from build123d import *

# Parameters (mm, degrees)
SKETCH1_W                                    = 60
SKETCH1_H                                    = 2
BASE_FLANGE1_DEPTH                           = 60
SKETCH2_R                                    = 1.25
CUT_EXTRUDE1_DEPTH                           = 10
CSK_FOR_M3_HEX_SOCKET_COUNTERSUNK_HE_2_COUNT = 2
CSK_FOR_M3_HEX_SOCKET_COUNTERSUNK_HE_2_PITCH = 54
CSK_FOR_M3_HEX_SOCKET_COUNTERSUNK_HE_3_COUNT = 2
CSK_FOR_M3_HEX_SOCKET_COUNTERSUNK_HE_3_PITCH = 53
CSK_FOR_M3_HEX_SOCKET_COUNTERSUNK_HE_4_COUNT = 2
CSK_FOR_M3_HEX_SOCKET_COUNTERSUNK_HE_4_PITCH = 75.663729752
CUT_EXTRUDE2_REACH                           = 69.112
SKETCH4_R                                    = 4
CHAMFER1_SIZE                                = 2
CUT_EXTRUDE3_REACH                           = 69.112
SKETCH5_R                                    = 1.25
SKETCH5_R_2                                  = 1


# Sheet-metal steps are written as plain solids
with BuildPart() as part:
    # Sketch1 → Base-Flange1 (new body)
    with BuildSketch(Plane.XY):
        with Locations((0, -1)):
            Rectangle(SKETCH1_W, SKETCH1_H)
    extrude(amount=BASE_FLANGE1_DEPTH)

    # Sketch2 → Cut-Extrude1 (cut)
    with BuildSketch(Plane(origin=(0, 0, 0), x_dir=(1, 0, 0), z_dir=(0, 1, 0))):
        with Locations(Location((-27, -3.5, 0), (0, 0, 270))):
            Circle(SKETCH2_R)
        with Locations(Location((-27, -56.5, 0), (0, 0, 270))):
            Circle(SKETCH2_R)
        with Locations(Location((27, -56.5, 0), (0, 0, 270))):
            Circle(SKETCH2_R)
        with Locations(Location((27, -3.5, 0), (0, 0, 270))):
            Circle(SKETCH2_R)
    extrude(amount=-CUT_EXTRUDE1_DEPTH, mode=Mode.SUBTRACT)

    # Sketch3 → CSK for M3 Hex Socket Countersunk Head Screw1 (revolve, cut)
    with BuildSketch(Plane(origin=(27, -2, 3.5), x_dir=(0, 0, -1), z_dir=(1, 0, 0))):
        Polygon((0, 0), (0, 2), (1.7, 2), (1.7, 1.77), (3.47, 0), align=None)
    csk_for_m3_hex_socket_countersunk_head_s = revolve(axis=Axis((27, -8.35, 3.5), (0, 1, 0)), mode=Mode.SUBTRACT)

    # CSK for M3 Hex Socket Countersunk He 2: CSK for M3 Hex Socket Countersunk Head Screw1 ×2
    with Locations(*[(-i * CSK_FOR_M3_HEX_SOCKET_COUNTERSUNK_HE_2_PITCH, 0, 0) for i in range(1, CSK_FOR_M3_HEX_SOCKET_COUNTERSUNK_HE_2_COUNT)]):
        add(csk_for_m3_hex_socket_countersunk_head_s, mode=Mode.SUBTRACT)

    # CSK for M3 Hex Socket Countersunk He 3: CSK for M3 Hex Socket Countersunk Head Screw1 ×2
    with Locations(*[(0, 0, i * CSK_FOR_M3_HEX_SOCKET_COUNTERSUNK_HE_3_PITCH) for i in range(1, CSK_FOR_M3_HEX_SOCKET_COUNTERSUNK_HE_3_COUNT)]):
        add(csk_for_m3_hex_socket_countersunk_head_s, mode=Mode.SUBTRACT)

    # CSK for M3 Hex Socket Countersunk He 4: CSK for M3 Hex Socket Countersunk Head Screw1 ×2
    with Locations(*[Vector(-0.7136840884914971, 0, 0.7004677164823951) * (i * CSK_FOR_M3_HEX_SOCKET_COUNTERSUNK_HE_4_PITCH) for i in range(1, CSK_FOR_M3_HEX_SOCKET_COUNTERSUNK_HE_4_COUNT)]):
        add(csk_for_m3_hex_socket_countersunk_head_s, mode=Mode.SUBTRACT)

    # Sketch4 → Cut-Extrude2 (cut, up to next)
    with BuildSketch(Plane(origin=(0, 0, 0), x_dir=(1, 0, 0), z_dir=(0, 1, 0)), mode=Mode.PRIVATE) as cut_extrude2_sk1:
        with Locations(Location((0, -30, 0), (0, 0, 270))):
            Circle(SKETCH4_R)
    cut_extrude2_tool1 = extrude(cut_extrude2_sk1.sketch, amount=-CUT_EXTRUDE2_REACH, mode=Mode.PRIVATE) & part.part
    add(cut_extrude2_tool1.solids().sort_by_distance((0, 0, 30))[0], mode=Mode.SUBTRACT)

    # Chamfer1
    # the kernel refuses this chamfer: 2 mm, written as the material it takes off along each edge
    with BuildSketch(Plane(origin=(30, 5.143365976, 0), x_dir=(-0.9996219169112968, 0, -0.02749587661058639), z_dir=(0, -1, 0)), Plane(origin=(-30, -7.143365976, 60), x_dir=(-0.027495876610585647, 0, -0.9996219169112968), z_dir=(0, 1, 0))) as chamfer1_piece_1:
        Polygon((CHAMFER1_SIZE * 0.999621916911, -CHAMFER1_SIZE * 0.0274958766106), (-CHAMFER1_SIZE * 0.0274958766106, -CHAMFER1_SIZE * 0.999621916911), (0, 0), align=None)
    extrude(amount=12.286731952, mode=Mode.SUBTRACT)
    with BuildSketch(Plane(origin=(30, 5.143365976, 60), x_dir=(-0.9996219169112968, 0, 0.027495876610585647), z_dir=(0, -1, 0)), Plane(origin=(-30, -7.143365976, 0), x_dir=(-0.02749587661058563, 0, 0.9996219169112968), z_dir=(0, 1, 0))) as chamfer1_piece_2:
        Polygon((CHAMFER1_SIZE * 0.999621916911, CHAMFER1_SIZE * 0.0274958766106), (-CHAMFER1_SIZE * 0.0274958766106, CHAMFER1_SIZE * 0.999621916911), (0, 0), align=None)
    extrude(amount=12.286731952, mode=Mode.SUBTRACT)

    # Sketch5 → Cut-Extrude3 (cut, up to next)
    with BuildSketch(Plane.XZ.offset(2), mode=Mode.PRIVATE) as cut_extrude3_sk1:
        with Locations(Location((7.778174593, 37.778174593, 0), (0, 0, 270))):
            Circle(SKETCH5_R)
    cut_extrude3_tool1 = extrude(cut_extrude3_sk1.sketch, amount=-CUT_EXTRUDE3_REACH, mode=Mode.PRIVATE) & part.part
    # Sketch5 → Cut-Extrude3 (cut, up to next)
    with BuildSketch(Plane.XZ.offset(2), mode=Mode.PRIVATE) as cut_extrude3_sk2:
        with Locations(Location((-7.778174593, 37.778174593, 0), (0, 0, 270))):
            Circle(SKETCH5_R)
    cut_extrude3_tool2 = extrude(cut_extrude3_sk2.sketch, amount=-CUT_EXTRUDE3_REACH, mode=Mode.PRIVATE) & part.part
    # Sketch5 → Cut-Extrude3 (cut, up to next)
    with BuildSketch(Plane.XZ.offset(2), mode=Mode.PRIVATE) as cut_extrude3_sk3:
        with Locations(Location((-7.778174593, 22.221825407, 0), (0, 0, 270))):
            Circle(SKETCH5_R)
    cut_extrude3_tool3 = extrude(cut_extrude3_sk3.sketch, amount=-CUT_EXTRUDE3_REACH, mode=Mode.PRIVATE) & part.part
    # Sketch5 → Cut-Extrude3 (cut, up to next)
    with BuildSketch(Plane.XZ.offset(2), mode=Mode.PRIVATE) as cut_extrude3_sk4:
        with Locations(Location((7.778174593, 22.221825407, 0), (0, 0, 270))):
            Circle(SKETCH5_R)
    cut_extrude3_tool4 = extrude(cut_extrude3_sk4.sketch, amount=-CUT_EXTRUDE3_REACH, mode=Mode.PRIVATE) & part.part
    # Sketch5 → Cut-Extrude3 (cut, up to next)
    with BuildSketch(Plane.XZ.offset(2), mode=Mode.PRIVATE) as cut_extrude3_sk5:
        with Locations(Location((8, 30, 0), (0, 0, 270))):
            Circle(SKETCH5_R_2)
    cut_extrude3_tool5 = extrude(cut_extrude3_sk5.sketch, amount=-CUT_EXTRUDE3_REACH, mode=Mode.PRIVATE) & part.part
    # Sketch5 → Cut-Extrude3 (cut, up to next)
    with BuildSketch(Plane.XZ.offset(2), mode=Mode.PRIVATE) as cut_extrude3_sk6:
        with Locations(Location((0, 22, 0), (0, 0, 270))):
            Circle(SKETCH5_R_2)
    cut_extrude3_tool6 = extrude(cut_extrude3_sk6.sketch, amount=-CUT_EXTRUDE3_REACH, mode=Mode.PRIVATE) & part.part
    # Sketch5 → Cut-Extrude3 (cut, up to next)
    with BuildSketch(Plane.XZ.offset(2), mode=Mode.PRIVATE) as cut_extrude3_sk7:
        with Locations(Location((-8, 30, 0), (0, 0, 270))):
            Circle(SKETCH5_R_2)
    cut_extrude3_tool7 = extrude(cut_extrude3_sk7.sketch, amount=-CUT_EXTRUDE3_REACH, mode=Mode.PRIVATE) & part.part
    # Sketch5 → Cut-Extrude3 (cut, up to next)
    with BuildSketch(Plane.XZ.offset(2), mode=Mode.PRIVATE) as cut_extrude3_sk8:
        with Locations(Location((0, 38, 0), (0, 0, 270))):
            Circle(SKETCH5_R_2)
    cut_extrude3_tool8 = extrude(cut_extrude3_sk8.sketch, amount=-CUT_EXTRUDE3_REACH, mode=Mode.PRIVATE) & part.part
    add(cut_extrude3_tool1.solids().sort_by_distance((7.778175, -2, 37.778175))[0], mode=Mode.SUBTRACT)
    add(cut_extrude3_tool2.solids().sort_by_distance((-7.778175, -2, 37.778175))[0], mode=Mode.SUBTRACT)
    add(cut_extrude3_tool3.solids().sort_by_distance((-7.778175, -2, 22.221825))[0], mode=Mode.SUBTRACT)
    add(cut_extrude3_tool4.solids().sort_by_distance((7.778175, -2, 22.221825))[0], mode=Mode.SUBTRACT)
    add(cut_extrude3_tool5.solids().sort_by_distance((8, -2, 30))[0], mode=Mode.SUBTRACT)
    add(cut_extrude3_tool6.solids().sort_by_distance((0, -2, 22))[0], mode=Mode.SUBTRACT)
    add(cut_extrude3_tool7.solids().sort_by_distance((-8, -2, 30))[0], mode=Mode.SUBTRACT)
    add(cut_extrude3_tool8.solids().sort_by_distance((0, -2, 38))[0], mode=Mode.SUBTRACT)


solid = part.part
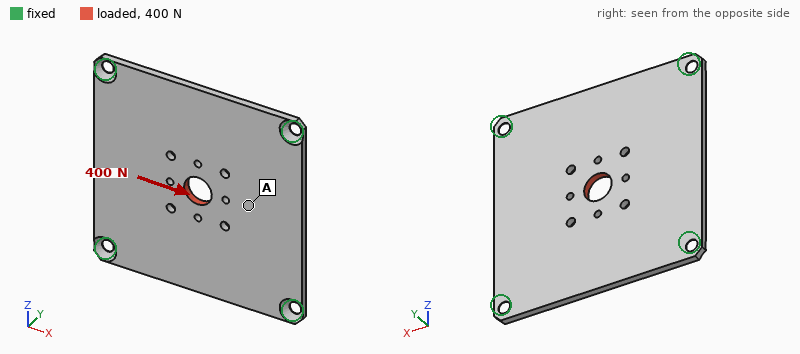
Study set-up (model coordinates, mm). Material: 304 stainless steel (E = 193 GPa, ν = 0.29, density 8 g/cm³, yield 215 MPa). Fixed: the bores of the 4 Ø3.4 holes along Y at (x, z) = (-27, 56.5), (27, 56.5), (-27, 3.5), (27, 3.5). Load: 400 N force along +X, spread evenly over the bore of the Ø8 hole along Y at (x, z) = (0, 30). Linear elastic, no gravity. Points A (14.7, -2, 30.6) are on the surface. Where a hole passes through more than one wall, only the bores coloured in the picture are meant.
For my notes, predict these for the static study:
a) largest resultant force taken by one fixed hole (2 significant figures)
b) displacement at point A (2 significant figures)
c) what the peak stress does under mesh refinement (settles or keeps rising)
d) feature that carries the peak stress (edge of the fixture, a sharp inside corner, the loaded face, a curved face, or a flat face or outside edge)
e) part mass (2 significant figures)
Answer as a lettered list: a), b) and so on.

a) 110 N
b) 1.5 µm
c) keeps rising
d) edge of the fixture
e) 55 g
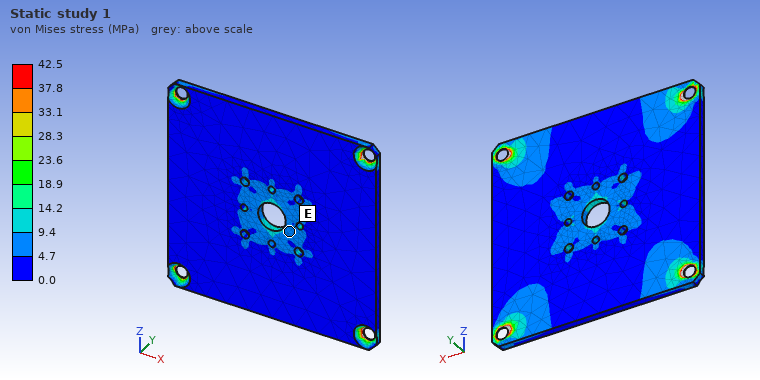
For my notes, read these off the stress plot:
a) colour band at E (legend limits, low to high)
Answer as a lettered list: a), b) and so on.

a) 4.7 to 9.4 MPa
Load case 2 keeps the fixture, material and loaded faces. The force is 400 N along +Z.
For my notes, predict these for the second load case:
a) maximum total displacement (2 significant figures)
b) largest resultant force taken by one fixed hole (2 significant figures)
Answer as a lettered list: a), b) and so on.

a) 1.7 µm
b) 110 N
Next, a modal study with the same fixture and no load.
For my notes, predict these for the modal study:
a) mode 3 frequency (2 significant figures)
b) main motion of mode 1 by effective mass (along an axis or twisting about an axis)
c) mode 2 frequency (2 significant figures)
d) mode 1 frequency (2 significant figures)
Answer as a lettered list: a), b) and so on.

a) 3400 Hz
b) along Y
c) 3300 Hz
d) 1900 Hz
